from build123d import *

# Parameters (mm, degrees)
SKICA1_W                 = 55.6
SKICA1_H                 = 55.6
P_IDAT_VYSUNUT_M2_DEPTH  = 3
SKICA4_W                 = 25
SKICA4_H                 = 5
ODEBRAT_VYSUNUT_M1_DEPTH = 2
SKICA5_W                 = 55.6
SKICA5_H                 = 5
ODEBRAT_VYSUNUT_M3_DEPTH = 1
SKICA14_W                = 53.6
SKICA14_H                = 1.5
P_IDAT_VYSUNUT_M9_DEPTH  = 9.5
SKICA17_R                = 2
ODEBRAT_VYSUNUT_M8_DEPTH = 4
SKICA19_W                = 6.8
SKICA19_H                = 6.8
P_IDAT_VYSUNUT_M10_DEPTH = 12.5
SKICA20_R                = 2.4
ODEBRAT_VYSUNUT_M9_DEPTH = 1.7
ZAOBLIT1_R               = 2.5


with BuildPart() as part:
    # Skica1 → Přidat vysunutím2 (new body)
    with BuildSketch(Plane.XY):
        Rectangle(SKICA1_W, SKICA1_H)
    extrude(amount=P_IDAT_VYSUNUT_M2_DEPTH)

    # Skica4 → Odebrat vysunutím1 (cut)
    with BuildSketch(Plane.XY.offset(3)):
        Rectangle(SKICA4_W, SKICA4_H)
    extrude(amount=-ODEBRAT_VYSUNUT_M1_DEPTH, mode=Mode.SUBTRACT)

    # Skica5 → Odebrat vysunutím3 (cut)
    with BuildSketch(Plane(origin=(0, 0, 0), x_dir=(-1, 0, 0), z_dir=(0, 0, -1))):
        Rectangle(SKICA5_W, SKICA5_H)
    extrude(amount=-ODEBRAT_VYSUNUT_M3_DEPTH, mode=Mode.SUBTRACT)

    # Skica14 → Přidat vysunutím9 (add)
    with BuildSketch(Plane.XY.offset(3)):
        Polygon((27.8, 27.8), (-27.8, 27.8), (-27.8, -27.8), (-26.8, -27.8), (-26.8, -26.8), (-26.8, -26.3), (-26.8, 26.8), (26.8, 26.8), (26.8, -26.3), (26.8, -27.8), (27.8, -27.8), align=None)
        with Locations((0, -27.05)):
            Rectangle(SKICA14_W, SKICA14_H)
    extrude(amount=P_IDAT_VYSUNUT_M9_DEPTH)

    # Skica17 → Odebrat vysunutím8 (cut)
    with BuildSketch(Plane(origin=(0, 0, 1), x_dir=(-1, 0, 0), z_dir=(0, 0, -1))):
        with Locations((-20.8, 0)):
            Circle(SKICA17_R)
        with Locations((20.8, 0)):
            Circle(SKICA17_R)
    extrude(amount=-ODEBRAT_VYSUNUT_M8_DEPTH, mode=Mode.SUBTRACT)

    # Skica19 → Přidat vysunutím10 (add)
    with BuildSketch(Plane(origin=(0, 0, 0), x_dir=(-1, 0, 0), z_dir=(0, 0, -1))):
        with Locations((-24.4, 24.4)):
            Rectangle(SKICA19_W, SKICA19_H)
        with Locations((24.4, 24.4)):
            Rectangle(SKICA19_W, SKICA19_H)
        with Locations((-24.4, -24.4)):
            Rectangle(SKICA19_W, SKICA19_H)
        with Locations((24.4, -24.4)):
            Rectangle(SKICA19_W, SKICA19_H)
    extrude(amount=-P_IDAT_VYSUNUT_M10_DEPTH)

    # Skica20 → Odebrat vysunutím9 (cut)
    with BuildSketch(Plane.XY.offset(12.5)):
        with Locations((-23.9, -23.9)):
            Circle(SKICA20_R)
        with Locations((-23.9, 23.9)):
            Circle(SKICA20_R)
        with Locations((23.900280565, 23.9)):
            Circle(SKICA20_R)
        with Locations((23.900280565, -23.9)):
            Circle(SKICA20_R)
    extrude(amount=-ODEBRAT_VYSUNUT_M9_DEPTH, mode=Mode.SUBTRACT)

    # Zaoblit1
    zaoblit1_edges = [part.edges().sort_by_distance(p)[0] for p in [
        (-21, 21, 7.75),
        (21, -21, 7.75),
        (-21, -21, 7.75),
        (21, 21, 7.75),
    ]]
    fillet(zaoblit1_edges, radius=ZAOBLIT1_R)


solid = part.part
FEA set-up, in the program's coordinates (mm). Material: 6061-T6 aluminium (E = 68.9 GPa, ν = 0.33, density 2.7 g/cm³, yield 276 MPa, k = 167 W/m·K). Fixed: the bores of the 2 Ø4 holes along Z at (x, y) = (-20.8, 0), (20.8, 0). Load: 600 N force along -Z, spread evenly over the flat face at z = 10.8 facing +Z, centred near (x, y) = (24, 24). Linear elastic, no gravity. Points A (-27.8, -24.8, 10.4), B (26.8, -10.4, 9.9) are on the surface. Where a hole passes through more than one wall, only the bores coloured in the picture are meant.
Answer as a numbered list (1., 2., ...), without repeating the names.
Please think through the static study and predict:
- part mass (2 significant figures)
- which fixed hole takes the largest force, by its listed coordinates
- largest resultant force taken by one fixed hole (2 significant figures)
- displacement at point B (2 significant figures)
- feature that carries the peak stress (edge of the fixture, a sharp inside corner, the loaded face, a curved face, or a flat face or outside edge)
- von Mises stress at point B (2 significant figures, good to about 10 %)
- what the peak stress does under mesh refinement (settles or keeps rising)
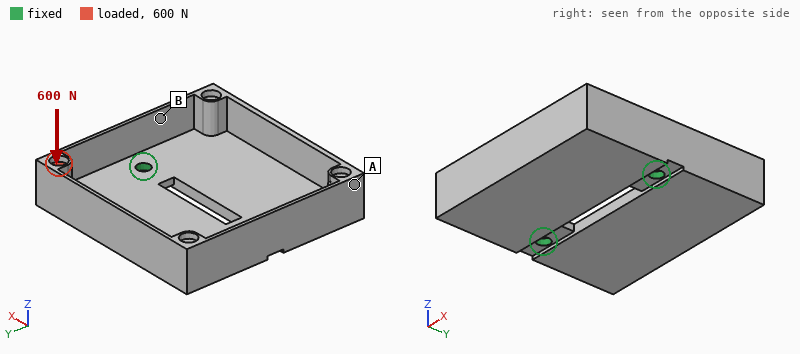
1. 33 g
2. (20.8, 0)
3. 600 N
4. 0.19 mm
5. edge of the fixture
6. 65 MPa
7. keeps rising
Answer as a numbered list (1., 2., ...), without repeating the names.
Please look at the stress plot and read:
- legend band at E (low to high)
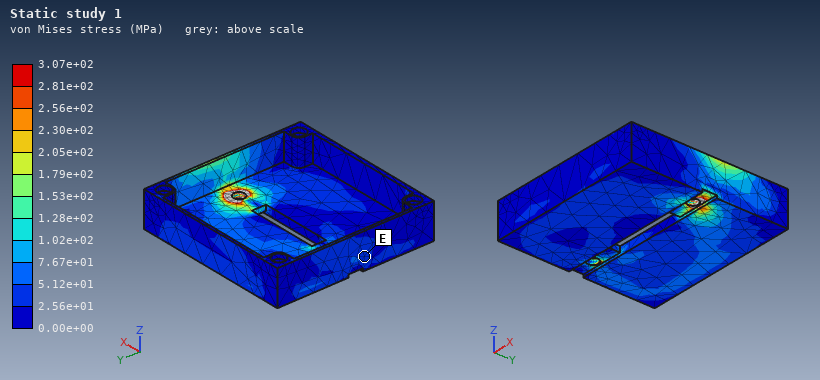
1. 2.56e+01 to 5.12e+01 MPa
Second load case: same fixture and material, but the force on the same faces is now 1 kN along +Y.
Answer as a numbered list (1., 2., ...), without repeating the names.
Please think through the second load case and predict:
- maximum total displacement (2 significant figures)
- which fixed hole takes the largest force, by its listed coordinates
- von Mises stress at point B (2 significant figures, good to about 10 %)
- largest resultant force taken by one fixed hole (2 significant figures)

1. 0.46 mm
2. (20.8, 0)
3. 38 MPa
4. 1.1 kN
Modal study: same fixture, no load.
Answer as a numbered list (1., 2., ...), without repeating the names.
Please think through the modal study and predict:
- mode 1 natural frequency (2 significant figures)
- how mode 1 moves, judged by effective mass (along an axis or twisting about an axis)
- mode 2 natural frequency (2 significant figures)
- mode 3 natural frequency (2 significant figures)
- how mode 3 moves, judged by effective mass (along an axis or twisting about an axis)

1. 1700 Hz
2. twisting about X
3. 2900 Hz
4. 3700 Hz
5. along Z
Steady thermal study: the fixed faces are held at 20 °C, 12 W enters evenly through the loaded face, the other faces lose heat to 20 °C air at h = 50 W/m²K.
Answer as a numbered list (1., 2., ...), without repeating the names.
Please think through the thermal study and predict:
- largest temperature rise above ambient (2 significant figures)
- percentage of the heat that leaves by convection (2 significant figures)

1. 34 K
2. 22 %
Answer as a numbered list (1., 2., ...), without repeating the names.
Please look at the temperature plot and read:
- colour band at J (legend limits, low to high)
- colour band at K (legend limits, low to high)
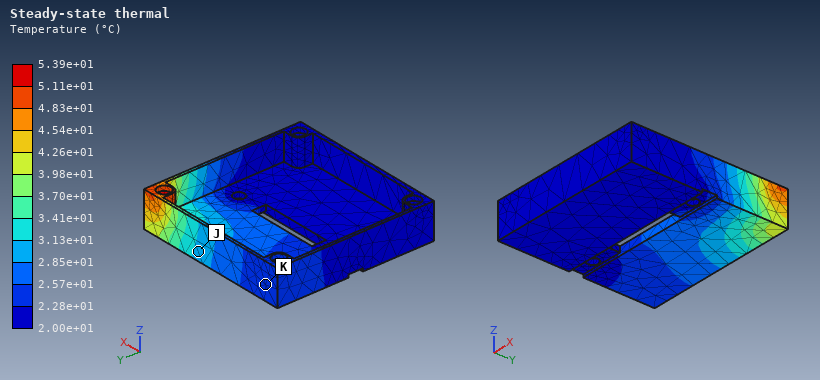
1. 2.85e+01 to 3.13e+01 °C
2. 2.28e+01 to 2.57e+01 °C
